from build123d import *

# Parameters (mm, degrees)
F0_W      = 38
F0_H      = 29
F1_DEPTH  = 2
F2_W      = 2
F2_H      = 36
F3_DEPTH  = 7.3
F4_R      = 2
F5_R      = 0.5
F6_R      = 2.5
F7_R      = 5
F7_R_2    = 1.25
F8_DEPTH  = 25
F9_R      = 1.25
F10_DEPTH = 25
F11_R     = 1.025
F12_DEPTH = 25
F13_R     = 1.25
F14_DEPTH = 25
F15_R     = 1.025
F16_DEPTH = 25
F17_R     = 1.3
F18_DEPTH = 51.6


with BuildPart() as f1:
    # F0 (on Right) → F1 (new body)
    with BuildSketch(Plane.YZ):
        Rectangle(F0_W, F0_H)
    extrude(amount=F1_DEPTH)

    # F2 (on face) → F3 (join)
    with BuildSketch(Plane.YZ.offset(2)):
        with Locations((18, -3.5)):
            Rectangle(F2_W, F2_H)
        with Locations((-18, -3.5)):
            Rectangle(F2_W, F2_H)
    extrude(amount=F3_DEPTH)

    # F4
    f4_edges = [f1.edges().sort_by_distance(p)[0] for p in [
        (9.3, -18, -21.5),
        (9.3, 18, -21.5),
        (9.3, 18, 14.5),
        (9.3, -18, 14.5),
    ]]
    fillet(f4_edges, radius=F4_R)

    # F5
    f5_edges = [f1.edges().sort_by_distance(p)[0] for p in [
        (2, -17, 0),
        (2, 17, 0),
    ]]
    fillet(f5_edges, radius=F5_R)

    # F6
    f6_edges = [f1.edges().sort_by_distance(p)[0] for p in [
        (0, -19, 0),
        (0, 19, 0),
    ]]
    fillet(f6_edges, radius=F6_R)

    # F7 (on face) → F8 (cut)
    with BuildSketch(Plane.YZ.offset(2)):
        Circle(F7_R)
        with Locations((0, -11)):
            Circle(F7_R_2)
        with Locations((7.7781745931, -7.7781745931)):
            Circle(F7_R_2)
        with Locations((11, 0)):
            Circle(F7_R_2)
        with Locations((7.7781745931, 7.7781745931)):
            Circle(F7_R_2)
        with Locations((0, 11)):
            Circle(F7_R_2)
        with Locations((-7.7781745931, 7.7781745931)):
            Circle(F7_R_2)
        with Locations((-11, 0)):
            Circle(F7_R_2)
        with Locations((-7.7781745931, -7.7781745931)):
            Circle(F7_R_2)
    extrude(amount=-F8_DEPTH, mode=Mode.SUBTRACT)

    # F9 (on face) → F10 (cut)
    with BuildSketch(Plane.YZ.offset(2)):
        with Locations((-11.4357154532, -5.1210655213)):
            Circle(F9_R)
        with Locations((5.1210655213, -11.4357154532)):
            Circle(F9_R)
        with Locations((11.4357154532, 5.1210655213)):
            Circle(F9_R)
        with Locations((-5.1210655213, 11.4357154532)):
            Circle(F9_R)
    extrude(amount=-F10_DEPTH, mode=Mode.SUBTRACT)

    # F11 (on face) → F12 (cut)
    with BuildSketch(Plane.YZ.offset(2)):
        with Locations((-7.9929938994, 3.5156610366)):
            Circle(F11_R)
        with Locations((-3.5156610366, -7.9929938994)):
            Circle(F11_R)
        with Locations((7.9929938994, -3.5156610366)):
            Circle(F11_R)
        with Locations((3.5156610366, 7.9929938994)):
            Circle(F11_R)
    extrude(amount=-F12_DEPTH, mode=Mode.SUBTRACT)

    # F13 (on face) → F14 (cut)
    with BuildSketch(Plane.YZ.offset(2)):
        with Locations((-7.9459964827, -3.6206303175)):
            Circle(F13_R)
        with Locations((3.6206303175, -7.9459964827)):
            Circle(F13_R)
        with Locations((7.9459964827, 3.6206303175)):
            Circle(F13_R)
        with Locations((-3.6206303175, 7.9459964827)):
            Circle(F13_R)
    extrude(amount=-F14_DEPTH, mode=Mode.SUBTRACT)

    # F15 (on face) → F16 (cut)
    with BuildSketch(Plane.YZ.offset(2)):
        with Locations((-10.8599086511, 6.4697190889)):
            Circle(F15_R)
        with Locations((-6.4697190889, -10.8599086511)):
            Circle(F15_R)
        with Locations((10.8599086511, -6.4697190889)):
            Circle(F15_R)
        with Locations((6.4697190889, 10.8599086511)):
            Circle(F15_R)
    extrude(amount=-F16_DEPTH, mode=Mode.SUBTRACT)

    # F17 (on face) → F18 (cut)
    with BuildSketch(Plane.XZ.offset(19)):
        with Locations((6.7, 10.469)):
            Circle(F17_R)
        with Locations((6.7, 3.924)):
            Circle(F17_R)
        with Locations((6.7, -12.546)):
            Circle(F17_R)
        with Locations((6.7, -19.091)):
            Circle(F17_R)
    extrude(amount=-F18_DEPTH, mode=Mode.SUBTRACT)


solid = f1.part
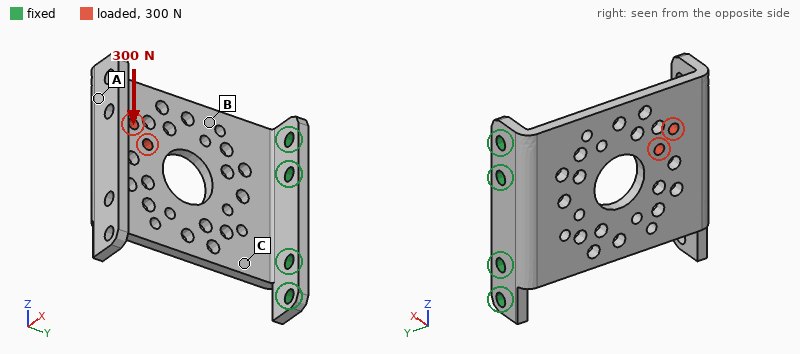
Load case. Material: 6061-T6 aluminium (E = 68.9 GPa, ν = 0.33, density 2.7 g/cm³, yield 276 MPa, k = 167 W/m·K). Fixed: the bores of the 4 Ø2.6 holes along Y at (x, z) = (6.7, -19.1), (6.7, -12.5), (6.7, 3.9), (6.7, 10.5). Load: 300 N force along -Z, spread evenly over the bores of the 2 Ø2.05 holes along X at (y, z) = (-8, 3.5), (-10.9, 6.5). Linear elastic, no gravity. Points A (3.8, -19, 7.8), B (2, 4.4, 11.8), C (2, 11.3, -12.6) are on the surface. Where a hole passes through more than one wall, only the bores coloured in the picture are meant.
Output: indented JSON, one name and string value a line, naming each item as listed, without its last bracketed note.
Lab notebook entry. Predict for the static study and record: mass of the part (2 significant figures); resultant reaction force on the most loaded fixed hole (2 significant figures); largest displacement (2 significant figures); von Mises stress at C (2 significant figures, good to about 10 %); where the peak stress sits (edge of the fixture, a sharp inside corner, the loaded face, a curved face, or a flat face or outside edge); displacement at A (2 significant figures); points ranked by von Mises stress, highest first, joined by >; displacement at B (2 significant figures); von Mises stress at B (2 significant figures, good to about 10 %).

{
  "mass of the part": "7.3 g",
  "resultant reaction force on the most loaded fixed hole": "340 N",
  "largest displacement": "0.18 mm",
  "von Mises stress at C": "58 MPa",
  "where the peak stress sits": "a sharp inside corner",
  "displacement at A": "0.14 mm",
  "points ranked by von Mises stress, highest first, joined by >": "C > B > A",
  "displacement at B": "0.071 mm",
  "von Mises stress at B": "38 MPa"
}
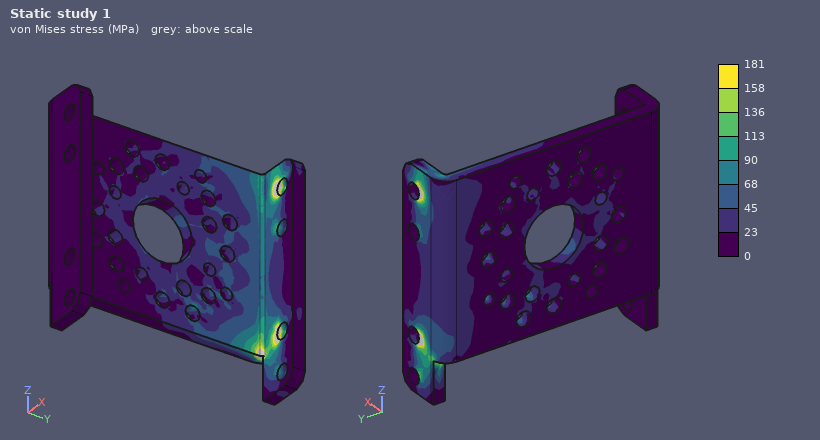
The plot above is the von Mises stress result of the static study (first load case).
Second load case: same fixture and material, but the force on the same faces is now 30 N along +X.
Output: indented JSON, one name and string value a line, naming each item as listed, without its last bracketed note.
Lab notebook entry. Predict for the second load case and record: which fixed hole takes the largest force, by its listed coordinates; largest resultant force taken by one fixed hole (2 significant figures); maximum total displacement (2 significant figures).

{
  "which fixed hole takes the largest force, by its listed coordinates": "(6.7, 3.9)",
  "largest resultant force taken by one fixed hole": "27 N",
  "maximum total displacement": "0.46 mm"
}
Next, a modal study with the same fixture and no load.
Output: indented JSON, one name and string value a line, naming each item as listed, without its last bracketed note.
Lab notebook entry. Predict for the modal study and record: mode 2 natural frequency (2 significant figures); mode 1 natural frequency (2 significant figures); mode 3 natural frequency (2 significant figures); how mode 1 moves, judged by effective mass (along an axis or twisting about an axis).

{
  "mode 2 natural frequency": "1900 Hz",
  "mode 1 natural frequency": "690 Hz",
  "mode 3 natural frequency": "4200 Hz",
  "how mode 1 moves, judged by effective mass": "along X"
}
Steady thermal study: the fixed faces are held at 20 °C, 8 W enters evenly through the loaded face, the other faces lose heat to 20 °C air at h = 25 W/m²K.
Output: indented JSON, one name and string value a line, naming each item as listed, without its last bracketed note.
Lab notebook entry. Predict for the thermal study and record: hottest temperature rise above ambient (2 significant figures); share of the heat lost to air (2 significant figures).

{
  "hottest temperature rise above ambient": "40 K",
  "share of the heat lost to air": "21 %"
}
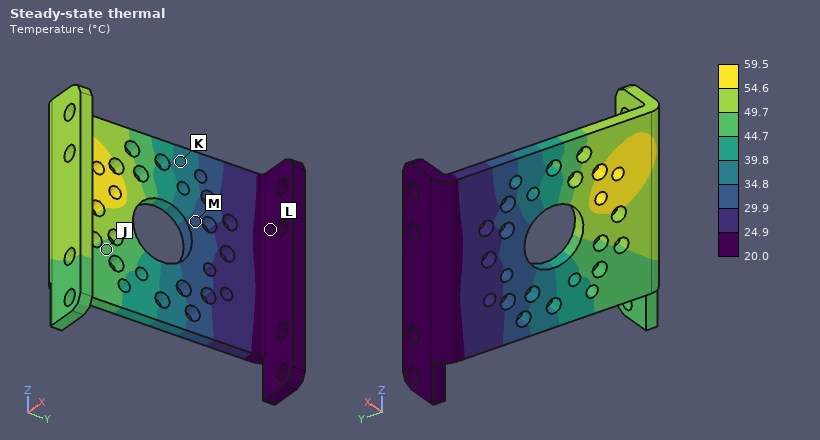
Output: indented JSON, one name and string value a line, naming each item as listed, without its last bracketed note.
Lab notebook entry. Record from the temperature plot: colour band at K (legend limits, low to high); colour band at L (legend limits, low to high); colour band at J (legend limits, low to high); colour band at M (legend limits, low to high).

{
  "colour band at K": "34.8 to 39.8 °C",
  "colour band at L": "20.0 to 24.9 °C",
  "colour band at J": "44.7 to 49.7 °C",
  "colour band at M": "29.9 to 34.8 °C"
}
